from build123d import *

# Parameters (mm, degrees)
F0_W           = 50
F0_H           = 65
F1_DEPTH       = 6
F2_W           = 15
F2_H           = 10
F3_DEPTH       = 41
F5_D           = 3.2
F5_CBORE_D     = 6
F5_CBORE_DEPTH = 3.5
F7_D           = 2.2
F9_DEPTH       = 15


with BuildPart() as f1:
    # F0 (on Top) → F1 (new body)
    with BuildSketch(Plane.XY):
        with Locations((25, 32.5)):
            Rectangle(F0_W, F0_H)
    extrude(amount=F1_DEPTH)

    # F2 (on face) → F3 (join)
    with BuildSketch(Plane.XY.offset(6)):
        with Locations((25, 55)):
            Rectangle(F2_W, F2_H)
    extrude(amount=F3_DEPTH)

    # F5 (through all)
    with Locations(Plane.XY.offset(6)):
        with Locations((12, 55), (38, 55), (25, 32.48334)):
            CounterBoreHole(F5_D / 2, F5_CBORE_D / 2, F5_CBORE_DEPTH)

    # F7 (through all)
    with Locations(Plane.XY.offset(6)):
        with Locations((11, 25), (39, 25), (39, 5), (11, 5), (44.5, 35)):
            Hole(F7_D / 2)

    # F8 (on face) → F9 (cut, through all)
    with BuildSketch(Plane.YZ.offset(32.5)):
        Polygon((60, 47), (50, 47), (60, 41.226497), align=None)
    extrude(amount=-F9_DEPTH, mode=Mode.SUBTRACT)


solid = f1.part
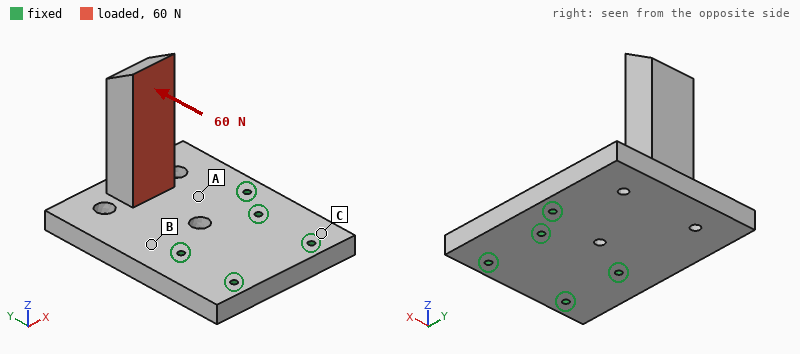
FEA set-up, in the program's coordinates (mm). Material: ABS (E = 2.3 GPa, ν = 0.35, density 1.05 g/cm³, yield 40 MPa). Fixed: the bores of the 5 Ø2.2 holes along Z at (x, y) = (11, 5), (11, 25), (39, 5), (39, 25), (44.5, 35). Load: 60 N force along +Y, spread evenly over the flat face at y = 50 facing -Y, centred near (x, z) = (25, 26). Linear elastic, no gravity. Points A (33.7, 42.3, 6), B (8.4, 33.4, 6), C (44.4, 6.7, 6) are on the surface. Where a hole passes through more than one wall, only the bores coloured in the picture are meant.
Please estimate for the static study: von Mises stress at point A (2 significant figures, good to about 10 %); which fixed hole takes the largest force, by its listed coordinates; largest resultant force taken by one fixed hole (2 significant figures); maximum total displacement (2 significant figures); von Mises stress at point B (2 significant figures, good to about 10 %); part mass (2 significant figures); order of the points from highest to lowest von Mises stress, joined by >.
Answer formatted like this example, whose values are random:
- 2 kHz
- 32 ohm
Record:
- 5.0 MPa
- (44.5, 35)
- 39 N
- 1.0 mm
- 3.9 MPa
- 26 g
- A > B > C
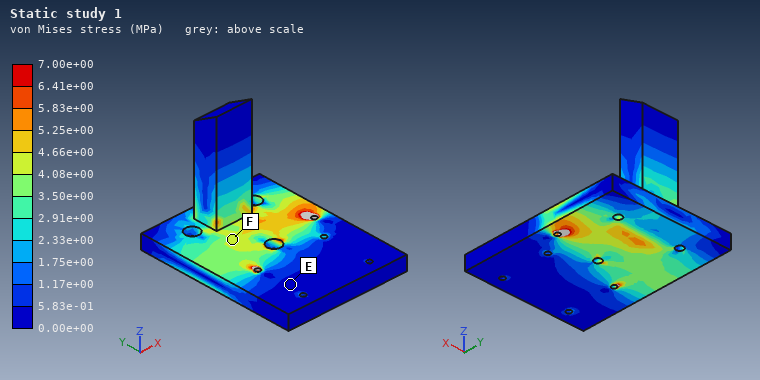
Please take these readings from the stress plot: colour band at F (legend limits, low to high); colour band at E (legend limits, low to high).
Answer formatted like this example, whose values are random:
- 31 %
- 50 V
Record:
- 4.08e+00 to 4.66e+00 MPa
- 0.00e+00 to 5.83e-01 MPa
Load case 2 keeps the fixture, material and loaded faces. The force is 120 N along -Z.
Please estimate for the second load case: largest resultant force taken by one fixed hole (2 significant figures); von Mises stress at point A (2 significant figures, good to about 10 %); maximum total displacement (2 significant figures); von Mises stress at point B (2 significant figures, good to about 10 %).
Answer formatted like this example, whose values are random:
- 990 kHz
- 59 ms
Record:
- 90 N
- 3.8 MPa
- 0.65 mm
- 4.8 MPa
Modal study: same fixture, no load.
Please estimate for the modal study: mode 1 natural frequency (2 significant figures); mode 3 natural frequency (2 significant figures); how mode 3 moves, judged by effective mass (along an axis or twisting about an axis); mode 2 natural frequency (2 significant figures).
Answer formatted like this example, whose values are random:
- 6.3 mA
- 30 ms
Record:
- 510 Hz
- 1400 Hz
- along Z
- 900 Hz
